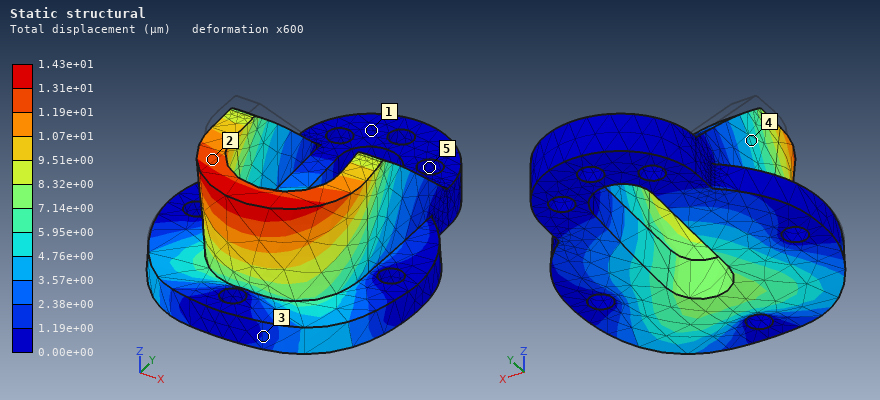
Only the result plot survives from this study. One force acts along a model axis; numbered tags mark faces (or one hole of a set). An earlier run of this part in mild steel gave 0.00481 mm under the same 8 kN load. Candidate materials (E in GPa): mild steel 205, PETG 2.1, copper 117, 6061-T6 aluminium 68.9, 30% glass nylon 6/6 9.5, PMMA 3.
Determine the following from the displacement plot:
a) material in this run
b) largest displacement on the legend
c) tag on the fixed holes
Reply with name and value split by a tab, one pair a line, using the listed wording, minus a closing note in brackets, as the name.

material in this run	6061-T6 aluminium
largest displacement on the legend	1.43e+01 µm
tag on the fixed holes	5
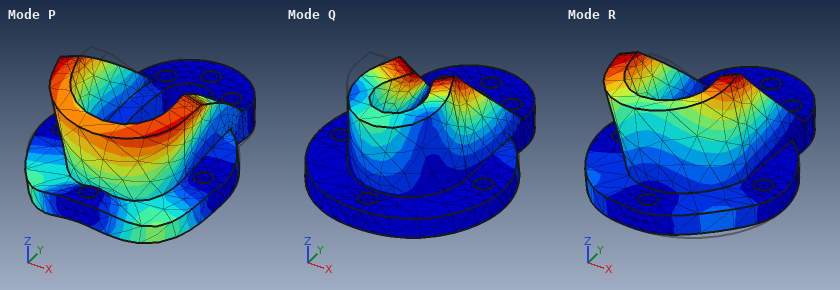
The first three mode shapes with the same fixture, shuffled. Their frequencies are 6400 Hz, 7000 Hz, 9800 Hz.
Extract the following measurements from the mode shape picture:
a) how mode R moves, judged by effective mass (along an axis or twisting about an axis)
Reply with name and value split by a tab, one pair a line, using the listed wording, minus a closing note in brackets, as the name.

how mode R moves, judged by effective mass	along X
